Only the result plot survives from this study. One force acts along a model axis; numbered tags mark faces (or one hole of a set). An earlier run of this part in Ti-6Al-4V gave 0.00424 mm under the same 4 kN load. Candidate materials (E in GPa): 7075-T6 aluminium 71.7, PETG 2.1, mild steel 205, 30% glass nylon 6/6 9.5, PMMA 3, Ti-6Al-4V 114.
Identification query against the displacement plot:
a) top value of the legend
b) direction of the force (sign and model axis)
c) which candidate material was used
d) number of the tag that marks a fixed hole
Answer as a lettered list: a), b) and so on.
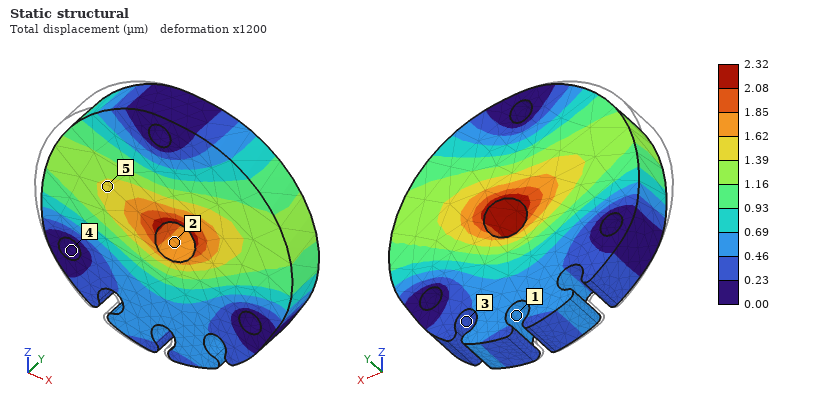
a) 2.32 µm
b) +X
c) mild steel
d) 4
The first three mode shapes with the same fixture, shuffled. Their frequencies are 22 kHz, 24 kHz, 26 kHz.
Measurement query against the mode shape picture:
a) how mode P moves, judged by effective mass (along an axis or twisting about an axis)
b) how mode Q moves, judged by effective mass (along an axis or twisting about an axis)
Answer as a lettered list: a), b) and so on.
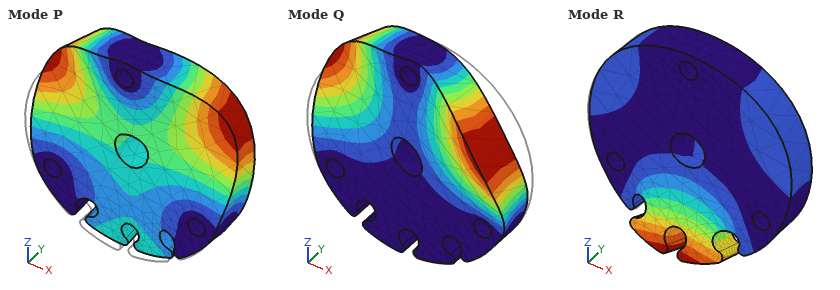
a) along Y
b) twisting about Z
